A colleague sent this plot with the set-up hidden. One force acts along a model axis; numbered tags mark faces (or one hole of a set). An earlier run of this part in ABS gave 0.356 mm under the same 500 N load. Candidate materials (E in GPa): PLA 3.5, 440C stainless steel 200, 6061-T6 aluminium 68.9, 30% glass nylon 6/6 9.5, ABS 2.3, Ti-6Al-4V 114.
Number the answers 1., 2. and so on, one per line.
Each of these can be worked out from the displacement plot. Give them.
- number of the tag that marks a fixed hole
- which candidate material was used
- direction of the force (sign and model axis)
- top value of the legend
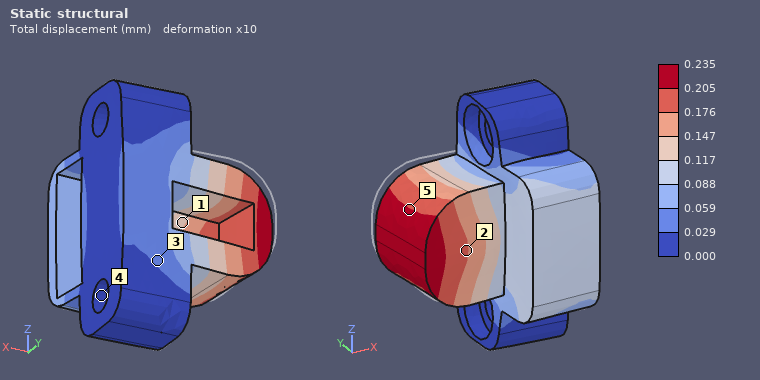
1. 4
2. PLA
3. -Y
4. 0.235 mm
